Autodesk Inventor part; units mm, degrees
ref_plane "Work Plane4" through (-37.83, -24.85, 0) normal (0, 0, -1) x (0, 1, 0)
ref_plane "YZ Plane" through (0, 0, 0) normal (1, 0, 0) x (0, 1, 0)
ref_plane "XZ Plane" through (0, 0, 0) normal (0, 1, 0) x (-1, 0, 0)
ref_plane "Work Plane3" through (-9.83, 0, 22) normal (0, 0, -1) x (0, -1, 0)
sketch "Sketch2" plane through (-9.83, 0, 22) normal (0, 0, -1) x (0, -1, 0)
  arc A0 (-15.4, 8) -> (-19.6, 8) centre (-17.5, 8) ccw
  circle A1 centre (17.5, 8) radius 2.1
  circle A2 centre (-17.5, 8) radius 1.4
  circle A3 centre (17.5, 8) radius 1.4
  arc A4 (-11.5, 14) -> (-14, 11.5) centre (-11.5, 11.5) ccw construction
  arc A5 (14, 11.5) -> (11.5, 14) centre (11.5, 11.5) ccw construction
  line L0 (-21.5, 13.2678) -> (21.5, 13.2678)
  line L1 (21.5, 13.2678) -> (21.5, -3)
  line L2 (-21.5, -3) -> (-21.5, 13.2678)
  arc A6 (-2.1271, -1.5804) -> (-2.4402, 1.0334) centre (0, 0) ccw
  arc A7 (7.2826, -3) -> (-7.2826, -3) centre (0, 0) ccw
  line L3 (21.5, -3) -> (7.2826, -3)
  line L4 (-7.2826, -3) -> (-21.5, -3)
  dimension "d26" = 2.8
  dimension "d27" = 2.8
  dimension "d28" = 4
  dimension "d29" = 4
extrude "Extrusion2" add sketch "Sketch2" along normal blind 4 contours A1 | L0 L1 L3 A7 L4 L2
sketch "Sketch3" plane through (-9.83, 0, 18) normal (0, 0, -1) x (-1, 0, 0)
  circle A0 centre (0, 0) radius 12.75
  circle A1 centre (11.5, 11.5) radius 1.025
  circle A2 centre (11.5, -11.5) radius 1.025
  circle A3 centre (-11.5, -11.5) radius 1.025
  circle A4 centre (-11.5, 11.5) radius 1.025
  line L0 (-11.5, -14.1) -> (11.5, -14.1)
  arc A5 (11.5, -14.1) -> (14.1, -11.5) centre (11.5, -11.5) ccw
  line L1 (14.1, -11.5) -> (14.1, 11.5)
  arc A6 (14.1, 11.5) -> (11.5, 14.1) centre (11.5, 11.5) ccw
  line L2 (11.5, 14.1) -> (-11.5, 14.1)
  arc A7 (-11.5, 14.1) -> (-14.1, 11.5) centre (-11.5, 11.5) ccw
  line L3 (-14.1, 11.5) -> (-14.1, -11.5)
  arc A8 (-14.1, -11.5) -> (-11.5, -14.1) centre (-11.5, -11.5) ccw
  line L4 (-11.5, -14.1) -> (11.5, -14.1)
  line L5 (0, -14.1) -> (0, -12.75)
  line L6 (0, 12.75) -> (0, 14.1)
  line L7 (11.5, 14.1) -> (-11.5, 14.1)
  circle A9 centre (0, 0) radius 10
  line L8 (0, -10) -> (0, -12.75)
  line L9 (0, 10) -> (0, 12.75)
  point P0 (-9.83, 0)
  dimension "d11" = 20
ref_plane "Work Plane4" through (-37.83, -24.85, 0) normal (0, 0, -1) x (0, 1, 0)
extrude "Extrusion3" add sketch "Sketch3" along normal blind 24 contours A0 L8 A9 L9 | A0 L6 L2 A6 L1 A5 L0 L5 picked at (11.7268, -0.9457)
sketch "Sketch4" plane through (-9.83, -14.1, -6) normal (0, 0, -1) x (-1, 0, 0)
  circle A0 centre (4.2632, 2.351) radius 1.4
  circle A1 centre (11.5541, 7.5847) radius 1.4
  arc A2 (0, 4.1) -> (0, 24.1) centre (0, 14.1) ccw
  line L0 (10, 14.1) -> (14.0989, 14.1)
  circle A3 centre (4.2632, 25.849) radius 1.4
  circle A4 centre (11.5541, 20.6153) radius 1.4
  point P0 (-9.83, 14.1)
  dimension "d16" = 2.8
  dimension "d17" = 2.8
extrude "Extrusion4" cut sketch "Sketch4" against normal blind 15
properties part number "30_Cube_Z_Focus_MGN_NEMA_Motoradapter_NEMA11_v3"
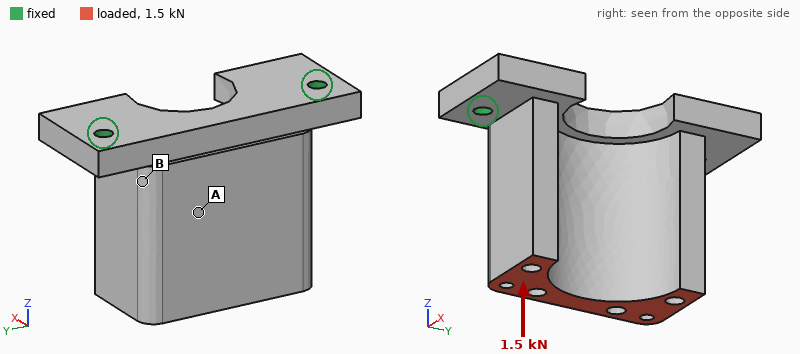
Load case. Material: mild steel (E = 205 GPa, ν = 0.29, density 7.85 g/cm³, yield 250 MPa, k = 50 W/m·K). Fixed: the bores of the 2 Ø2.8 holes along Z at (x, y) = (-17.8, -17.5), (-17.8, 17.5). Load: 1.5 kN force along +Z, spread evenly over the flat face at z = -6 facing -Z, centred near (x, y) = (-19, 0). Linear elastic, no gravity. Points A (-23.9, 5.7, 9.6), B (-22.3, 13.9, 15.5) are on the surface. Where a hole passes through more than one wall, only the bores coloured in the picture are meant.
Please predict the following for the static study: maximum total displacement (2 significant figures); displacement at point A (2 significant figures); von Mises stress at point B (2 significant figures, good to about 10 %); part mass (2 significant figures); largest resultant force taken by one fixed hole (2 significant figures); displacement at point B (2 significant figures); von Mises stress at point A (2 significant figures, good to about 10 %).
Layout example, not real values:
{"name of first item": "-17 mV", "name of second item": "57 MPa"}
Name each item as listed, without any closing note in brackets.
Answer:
{"maximum total displacement": "8.5 µm", "displacement at point A": "5.3 µm", "von Mises stress at point B": "30 MPa", "part mass": "58 g", "largest resultant force taken by one fixed hole": "790 N", "displacement at point B": "3.4 µm", "von Mises stress at point A": "8.5 MPa"}
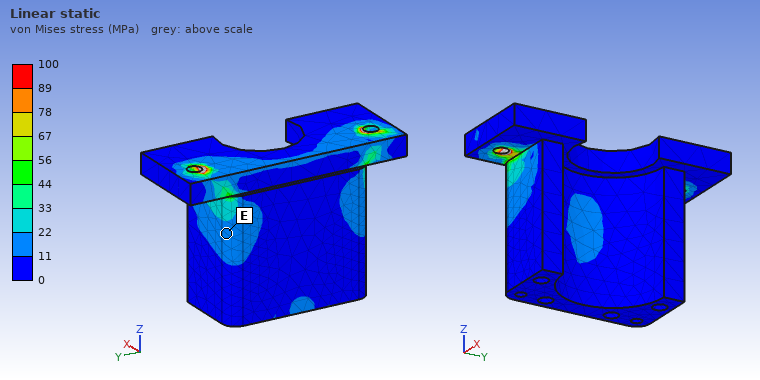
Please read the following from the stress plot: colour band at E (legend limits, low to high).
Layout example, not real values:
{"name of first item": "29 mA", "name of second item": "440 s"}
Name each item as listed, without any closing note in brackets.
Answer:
{"colour band at E": "11 to 22 MPa"}
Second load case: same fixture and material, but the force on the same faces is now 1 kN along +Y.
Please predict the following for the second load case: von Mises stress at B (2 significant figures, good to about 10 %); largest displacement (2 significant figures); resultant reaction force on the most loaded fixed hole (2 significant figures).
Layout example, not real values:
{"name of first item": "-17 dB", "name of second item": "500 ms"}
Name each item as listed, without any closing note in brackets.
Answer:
{"von Mises stress at B": "34 MPa", "largest displacement": "15 µm", "resultant reaction force on the most loaded fixed hole": "980 N"}
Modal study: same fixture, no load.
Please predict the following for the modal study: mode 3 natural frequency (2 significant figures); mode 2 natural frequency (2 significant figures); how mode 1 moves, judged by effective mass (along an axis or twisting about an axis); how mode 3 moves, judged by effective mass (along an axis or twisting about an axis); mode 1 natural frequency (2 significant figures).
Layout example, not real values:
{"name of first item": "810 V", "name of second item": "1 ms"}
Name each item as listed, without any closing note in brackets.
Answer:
{"mode 3 natural frequency": "15 kHz", "mode 2 natural frequency": "10 kHz", "how mode 1 moves, judged by effective mass": "along X", "how mode 3 moves, judged by effective mass": "along Y", "mode 1 natural frequency": "4200 Hz"}
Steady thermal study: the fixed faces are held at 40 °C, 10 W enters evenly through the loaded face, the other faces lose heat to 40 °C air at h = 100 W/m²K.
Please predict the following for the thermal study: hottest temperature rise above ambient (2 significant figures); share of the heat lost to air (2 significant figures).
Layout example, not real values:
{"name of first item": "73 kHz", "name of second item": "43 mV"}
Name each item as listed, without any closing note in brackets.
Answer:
{"hottest temperature rise above ambient": "23 K", "share of the heat lost to air": "50 %"}
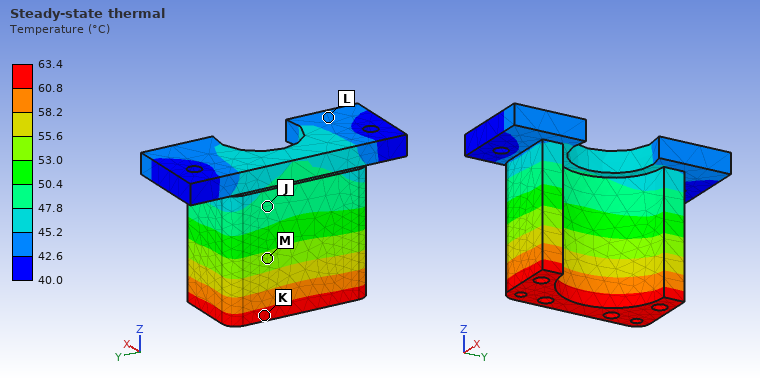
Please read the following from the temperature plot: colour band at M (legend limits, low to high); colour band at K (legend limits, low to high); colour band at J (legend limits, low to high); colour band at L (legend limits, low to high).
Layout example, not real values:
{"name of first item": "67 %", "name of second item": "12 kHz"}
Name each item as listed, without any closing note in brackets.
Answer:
{"colour band at M": "53.0 to 55.6 °C", "colour band at K": "60.8 to 63.4 °C", "colour band at J": "47.8 to 50.4 °C", "colour band at L": "42.6 to 45.2 °C"}
